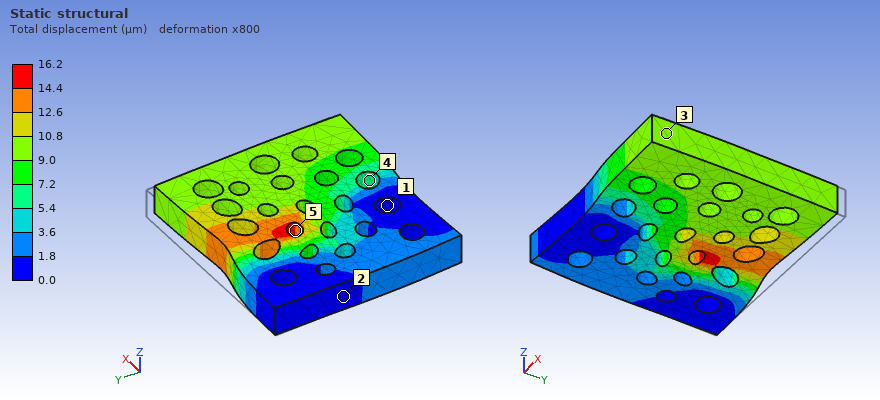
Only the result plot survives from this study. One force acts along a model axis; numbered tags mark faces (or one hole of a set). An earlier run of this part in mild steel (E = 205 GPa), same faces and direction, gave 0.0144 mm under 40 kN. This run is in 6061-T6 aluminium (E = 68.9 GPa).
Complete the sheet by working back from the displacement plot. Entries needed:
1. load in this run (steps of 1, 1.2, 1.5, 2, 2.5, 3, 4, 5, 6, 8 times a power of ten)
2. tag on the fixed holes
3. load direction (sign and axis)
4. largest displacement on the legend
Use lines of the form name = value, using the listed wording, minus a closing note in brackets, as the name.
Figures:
load in this run = 15 kN
tag on the fixed holes = 1
load direction = -Y
largest displacement on the legend = 16.2 µm
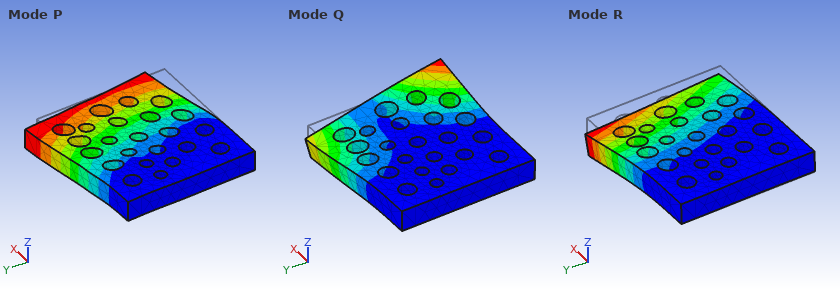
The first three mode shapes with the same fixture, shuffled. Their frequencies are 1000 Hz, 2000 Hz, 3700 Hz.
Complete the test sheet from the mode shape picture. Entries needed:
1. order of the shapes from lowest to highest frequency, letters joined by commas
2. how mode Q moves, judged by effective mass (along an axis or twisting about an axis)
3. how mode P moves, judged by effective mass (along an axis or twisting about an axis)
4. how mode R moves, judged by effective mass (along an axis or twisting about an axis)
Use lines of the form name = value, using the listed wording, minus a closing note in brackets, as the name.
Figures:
order of the shapes from lowest to highest frequency, letters joined by commas = R, Q, P
how mode Q moves, judged by effective mass = twisting about X
how mode P moves, judged by effective mass = along Y
how mode R moves, judged by effective mass = along Z
